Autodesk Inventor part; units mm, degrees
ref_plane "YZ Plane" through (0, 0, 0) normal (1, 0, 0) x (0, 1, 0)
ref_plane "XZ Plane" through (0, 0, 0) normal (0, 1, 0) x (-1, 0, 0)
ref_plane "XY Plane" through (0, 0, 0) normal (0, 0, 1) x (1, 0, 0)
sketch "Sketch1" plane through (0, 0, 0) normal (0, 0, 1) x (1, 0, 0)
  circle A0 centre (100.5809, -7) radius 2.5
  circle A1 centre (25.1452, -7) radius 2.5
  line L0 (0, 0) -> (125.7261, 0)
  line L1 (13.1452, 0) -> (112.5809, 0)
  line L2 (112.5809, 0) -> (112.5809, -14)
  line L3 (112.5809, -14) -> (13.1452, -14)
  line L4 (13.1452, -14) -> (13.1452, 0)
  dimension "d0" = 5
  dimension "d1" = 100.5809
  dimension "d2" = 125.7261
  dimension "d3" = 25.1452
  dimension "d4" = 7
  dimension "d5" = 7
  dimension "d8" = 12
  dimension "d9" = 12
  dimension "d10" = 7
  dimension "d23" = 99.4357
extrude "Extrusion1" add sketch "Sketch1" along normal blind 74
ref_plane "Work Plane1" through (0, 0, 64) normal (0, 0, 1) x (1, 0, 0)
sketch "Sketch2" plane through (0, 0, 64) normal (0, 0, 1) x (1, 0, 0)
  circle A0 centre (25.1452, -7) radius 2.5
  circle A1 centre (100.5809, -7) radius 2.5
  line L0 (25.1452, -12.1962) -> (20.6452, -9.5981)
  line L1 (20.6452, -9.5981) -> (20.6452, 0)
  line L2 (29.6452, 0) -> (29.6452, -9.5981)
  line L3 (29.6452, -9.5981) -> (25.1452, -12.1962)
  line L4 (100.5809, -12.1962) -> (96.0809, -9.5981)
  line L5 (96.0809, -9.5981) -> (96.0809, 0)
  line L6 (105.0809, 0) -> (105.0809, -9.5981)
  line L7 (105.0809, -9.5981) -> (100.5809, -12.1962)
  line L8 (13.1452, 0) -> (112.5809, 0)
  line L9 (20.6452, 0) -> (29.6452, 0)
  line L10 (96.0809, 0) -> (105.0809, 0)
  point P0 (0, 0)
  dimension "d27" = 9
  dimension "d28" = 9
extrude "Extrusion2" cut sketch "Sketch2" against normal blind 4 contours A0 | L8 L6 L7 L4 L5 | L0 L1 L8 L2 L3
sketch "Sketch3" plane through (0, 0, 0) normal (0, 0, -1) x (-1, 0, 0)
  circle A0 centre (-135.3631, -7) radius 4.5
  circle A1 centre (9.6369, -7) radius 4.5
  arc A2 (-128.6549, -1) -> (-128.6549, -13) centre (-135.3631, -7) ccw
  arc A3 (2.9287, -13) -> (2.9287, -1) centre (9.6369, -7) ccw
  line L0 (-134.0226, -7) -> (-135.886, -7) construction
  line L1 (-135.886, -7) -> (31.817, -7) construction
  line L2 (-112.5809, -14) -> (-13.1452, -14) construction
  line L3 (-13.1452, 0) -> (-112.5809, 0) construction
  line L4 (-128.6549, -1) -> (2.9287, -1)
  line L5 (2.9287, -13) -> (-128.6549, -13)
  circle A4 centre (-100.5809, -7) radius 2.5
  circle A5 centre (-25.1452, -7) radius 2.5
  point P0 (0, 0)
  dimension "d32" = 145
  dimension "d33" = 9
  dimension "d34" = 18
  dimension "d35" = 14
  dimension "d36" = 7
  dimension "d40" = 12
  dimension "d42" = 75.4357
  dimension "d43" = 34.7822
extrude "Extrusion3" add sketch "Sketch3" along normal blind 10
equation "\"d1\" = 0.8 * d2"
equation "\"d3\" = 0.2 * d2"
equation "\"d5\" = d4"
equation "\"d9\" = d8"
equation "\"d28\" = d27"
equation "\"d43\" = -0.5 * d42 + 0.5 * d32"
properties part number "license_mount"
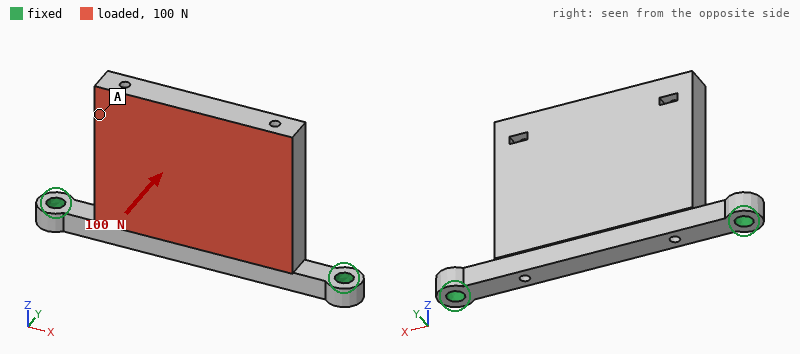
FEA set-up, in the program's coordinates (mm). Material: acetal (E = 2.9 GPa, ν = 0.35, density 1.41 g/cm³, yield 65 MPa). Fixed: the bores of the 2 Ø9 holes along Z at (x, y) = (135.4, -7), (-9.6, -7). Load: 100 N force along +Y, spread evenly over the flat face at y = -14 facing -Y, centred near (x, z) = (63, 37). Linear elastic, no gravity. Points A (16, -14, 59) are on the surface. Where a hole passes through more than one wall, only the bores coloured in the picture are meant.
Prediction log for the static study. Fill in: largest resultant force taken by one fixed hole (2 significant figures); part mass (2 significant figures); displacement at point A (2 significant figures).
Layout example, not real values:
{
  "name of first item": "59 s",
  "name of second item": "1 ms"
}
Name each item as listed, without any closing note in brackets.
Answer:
{
  "largest resultant force taken by one fixed hole": "50 N",
  "part mass": "170 g",
  "displacement at point A": "1.6 mm"
}
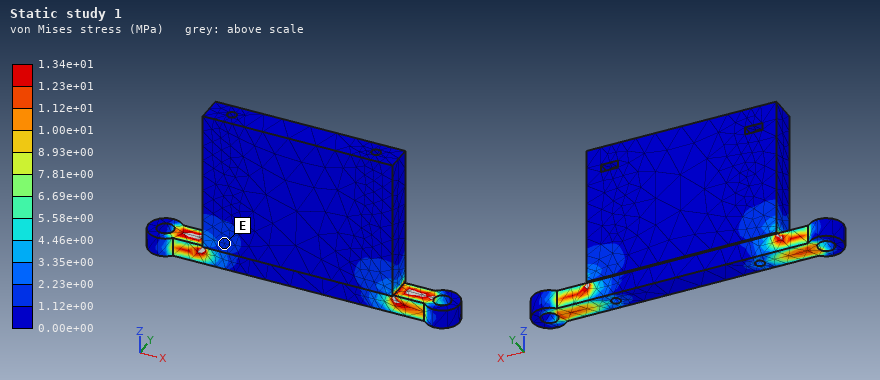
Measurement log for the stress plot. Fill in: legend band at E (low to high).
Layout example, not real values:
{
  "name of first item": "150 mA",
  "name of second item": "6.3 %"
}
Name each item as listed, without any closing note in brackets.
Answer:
{
  "legend band at E": "1.12e+00 to 2.23e+00 MPa"
}
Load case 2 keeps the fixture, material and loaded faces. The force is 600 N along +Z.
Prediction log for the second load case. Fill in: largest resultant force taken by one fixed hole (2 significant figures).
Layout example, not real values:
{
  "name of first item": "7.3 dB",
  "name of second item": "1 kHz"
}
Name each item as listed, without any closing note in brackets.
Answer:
{
  "largest resultant force taken by one fixed hole": "350 N"
}
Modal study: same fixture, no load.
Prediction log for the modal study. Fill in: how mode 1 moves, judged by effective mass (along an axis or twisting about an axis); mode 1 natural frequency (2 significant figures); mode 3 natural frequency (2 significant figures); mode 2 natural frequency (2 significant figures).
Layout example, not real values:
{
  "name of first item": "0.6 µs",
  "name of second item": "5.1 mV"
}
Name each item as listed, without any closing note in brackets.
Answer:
{
  "how mode 1 moves, judged by effective mass": "along Y",
  "mode 1 natural frequency": "120 Hz",
  "mode 3 natural frequency": "710 Hz",
  "mode 2 natural frequency": "700 Hz"
}
